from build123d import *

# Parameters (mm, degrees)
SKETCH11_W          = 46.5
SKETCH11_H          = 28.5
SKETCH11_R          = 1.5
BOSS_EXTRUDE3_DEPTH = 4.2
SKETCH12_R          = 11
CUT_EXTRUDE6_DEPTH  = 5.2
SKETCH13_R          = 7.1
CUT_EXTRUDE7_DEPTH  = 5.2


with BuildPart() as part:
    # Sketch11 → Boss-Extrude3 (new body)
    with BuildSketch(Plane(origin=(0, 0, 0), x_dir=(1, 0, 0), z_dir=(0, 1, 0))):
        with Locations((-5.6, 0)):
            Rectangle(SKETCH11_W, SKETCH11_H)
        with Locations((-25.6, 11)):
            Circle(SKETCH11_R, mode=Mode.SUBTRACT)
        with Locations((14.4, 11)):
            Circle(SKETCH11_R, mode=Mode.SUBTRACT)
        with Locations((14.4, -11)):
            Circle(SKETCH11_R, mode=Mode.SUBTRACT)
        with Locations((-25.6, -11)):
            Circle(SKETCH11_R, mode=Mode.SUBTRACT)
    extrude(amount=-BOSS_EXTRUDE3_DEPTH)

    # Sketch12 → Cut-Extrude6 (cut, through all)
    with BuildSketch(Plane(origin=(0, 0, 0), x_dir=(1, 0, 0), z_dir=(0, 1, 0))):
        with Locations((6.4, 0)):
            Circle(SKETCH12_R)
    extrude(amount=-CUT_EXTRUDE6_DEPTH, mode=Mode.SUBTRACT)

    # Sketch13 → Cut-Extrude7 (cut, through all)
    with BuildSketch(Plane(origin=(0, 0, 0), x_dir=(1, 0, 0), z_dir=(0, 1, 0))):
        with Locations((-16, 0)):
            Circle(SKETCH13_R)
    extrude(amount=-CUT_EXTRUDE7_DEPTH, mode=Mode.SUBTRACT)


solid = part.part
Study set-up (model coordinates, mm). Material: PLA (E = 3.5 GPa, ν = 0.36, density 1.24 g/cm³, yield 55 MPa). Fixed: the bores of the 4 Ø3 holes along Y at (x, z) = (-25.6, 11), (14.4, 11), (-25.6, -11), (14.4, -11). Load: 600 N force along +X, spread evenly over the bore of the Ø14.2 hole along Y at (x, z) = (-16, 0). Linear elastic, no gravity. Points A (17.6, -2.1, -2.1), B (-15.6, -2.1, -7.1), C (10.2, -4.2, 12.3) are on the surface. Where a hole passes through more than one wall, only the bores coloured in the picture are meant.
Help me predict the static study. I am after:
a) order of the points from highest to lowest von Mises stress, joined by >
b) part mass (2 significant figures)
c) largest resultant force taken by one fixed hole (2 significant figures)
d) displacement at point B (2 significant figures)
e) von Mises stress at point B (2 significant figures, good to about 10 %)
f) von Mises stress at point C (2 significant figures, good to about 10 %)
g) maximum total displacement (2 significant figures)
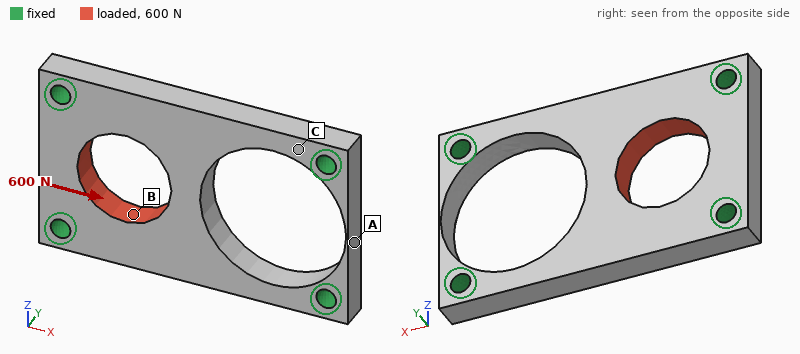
B > C > A
4.0 g
260 N
23 µm
9.0 MPa
3.7 MPa
52 µm
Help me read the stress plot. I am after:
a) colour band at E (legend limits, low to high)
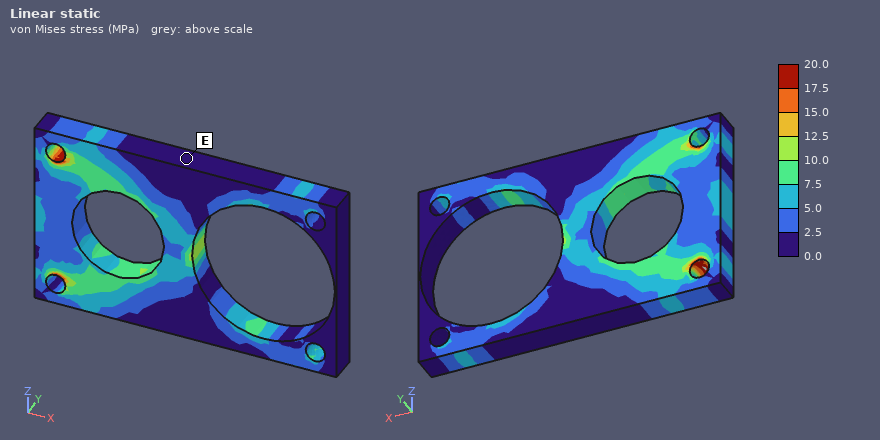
0.0 to 2.5 MPa
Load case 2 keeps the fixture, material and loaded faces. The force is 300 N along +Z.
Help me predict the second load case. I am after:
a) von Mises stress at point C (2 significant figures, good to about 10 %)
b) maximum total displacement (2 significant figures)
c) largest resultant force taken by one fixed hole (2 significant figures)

1.8 MPa
68 µm
150 N
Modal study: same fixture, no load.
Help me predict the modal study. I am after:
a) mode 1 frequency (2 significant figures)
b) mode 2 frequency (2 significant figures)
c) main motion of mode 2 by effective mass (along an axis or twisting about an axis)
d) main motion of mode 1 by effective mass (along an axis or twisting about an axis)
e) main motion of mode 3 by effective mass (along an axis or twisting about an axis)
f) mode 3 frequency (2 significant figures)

3700 Hz
5000 Hz
twisting about X
along Y
along Z
5900 Hz
